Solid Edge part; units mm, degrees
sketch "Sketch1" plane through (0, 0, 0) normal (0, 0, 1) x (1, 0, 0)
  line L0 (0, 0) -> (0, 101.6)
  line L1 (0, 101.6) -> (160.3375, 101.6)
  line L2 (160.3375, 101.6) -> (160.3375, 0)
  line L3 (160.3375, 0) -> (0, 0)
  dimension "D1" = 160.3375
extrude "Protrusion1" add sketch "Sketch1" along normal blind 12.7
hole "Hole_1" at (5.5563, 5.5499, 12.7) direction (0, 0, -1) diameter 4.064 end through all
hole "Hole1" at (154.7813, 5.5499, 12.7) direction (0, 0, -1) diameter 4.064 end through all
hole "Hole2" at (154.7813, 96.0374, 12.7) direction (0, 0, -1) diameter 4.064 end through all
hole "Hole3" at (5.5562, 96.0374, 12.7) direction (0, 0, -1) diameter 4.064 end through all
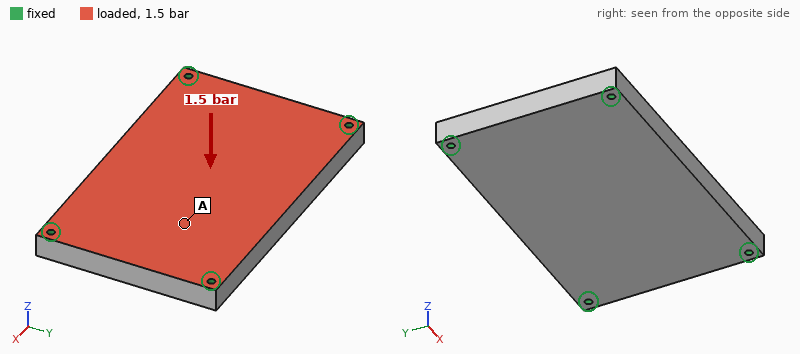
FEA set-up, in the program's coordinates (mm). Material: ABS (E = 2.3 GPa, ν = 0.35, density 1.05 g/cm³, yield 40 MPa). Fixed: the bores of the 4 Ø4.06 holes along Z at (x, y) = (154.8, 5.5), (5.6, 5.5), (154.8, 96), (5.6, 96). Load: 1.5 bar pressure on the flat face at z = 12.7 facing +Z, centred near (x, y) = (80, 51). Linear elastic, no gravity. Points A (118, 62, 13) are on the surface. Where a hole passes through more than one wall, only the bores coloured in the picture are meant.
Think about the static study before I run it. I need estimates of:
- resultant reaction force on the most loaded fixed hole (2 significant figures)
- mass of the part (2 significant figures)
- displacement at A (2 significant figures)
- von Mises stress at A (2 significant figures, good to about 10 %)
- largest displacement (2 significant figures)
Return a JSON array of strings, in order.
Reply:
["610 N", "220 g", "0.72 mm", "3.8 MPa", "1.0 mm"]
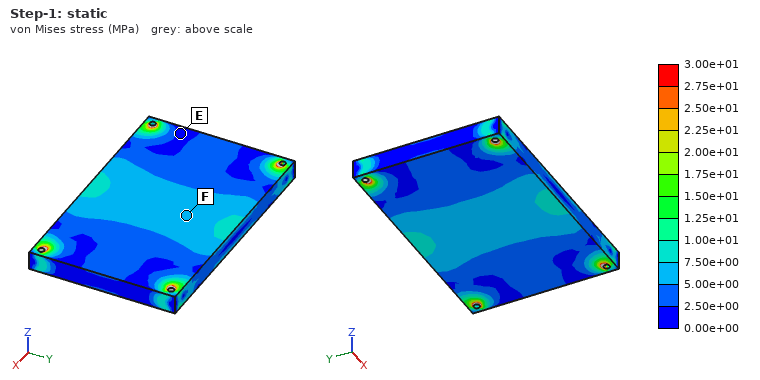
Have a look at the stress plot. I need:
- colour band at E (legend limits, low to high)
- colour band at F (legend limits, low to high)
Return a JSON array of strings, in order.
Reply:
["0.00e+00 to 2.50e+00 MPa", "5.00e+00 to 7.50e+00 MPa"]
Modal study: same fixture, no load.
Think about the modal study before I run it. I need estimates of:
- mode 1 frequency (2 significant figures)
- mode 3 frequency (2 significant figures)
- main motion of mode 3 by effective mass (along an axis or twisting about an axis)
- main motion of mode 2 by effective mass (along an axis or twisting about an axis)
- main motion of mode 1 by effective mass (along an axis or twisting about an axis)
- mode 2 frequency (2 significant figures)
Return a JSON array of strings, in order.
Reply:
["600 Hz", "1500 Hz", "twisting about Y", "twisting about X", "along Z", "1000 Hz"]
